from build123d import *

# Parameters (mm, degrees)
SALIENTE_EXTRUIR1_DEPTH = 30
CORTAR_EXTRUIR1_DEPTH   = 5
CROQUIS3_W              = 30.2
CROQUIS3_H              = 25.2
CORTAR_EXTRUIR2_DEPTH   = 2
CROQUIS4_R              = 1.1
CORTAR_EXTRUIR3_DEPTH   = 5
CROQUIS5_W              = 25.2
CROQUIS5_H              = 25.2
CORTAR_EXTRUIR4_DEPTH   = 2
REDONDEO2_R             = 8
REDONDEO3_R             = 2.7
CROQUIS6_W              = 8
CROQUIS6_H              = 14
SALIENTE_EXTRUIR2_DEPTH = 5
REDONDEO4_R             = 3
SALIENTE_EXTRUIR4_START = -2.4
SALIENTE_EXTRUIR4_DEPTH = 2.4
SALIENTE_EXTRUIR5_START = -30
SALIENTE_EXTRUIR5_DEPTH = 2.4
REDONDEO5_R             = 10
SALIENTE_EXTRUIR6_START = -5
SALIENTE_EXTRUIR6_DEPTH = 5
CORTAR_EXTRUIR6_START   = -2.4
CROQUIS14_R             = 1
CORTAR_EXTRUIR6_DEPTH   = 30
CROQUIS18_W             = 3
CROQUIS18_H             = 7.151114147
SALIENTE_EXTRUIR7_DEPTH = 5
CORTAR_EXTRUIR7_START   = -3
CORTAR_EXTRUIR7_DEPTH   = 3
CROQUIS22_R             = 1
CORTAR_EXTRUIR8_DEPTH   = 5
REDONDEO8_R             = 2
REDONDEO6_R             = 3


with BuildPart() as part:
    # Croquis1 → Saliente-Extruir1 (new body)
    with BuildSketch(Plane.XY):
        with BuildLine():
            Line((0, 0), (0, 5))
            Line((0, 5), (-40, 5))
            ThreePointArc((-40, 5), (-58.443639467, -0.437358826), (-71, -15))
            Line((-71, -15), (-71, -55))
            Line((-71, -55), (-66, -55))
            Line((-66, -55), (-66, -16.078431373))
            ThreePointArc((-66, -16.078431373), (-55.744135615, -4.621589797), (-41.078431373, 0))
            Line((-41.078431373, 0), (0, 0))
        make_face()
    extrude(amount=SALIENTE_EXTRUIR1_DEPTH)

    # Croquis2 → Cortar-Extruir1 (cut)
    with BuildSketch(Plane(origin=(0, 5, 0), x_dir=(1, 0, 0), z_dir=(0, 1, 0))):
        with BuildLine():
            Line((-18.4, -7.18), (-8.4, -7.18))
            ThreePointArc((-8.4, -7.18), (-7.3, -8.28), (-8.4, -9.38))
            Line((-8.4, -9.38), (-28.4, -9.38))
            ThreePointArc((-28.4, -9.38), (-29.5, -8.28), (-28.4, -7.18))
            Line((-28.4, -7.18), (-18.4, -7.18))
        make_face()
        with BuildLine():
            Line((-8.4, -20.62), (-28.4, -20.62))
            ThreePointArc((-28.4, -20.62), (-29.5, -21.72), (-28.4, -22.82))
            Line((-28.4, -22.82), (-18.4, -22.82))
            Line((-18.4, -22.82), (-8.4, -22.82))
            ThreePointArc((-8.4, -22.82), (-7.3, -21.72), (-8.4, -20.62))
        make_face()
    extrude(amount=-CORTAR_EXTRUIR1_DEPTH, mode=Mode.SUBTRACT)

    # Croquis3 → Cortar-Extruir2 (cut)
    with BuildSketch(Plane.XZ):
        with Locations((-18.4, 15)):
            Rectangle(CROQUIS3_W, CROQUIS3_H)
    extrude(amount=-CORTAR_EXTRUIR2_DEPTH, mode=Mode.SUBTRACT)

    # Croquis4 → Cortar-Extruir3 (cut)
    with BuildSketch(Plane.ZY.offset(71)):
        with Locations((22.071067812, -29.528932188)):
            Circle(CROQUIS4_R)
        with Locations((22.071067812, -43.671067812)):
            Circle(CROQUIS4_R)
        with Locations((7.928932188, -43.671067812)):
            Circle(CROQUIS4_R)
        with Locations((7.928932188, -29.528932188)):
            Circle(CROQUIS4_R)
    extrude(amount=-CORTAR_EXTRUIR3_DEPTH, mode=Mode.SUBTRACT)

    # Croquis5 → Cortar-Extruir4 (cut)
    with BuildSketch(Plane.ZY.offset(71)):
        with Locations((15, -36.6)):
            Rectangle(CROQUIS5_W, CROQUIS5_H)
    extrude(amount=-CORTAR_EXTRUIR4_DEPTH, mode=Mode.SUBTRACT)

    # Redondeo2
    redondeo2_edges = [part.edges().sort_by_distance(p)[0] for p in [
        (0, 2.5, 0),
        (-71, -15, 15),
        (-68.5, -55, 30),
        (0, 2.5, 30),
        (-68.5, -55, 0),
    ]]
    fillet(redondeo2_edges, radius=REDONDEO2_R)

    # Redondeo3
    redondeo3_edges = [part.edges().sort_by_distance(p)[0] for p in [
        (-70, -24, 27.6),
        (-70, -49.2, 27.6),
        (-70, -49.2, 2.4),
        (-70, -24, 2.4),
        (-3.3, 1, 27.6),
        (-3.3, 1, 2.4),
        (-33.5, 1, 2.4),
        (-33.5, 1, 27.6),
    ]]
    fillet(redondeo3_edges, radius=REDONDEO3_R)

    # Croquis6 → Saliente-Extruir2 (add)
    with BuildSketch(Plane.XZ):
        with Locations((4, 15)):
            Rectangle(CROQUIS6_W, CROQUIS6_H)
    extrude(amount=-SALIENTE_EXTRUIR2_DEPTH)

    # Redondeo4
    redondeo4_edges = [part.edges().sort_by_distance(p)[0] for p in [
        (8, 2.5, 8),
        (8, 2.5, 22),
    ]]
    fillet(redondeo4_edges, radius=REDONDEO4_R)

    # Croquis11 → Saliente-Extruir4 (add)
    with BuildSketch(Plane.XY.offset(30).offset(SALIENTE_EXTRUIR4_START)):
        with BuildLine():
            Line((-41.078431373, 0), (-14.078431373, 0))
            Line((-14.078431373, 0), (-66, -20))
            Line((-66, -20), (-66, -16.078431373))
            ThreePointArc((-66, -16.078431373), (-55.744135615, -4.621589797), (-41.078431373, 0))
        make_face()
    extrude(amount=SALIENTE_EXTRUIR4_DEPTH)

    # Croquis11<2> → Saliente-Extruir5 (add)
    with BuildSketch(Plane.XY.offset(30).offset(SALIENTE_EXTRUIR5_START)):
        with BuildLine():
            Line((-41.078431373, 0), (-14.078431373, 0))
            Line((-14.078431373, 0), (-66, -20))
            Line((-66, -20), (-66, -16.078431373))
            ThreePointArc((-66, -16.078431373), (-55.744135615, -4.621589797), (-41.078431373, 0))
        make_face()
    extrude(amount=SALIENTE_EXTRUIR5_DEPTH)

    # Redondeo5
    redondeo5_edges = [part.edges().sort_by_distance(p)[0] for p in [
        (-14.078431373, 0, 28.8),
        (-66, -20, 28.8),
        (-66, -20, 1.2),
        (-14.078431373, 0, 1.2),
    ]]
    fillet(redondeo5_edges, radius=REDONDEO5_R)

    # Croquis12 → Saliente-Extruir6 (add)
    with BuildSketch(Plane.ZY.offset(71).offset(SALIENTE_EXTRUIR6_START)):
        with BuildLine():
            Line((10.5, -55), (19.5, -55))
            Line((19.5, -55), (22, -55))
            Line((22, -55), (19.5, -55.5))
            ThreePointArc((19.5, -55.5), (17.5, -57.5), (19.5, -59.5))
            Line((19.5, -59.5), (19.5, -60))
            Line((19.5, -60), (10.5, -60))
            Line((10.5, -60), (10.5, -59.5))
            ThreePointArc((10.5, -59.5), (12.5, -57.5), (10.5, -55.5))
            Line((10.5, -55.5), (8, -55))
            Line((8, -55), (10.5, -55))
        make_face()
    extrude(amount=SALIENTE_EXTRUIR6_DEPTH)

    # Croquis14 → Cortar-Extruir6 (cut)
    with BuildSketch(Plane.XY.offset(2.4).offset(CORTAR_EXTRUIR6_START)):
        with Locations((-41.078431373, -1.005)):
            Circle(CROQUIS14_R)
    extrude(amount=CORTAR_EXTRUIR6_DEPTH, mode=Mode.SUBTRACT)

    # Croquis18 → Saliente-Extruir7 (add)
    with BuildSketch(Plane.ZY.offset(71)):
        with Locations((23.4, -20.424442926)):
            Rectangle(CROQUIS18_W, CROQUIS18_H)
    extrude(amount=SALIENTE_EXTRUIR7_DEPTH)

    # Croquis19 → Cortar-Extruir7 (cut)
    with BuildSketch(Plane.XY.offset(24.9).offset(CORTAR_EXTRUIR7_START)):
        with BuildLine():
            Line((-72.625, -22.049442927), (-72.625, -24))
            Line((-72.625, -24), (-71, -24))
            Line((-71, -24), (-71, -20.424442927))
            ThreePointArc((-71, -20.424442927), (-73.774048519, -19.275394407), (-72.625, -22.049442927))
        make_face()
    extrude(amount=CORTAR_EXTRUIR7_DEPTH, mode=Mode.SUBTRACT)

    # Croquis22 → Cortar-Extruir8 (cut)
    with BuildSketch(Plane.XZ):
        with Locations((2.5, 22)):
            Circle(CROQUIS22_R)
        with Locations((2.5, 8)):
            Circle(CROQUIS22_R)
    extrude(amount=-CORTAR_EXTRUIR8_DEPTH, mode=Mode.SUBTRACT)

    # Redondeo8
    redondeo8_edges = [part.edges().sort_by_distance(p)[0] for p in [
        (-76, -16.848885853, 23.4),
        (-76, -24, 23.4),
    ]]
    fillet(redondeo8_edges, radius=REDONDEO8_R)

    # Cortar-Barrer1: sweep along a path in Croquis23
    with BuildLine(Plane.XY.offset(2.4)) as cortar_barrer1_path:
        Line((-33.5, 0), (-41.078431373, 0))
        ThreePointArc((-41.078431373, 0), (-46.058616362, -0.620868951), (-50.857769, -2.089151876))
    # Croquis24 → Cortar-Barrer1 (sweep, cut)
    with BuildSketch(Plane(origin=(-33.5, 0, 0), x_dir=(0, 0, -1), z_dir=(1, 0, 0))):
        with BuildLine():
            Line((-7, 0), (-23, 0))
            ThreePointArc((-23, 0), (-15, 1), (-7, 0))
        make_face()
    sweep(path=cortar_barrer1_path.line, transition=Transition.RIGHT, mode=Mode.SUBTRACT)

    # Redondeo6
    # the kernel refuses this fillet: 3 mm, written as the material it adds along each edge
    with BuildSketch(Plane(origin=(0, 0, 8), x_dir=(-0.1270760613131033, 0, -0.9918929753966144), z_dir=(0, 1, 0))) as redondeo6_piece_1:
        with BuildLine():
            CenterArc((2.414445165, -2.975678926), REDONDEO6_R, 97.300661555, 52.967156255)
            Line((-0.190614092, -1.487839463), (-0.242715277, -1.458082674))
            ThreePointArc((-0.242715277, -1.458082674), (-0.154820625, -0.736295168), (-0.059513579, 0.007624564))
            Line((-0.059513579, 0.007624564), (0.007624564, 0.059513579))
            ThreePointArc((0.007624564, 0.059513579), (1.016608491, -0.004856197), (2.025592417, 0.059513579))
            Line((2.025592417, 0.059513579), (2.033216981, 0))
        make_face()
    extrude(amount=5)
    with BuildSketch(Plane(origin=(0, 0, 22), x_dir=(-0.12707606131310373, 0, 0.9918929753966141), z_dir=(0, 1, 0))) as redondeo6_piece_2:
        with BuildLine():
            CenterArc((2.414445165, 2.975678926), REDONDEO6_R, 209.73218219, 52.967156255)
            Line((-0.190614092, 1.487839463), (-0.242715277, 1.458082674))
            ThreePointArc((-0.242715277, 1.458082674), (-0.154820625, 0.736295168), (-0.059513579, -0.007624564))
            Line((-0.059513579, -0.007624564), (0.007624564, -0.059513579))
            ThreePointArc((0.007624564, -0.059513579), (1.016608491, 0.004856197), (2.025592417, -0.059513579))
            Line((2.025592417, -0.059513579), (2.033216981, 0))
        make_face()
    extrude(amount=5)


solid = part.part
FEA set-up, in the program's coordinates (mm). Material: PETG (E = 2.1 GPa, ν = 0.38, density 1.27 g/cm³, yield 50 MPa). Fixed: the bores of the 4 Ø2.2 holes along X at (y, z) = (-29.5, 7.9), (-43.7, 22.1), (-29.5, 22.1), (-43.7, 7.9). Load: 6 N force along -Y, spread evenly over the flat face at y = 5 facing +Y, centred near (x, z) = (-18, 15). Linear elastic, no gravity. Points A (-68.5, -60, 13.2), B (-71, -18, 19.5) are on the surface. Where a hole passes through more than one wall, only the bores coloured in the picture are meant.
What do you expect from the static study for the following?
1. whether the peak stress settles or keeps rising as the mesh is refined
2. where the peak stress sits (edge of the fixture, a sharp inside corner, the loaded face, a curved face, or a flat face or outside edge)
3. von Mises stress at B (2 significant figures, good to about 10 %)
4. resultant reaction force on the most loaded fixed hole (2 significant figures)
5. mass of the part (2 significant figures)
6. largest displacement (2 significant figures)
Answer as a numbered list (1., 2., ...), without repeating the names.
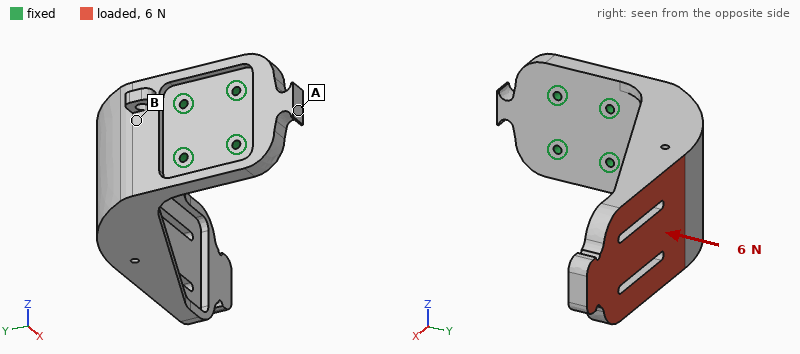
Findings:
1. keeps rising
2. edge of the fixture
3. 1.1 MPa
4. 8.5 N
5. 21 g
6. 1.2 mm
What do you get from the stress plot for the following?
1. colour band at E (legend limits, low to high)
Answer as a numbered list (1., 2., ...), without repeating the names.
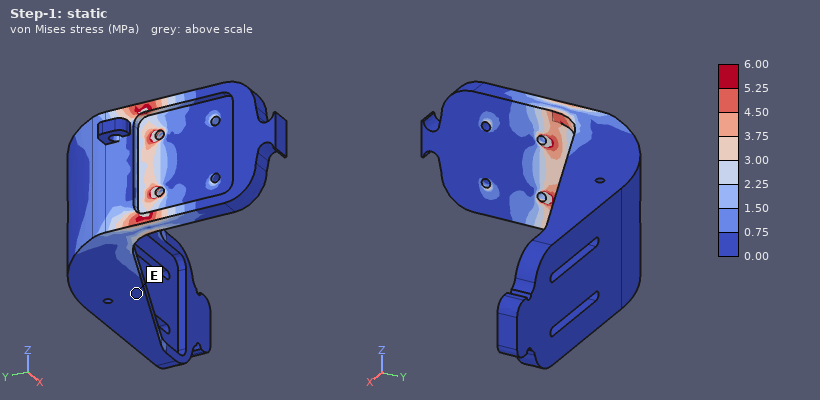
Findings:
1. 0.00 to 0.75 MPa
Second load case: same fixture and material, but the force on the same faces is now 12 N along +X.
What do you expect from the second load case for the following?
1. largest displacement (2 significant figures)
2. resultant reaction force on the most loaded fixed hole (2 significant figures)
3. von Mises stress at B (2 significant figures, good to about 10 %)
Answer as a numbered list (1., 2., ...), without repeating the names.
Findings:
1. 1.3 mm
2. 15 N
3. 1.1 MPa
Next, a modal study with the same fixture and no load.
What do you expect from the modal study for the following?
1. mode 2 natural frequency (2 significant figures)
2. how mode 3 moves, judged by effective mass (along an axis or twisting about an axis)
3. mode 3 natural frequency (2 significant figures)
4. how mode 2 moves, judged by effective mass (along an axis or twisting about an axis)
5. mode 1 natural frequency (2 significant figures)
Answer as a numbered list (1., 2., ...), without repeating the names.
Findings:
1. 250 Hz
2. along X
3. 810 Hz
4. along Z
5. 150 Hz
